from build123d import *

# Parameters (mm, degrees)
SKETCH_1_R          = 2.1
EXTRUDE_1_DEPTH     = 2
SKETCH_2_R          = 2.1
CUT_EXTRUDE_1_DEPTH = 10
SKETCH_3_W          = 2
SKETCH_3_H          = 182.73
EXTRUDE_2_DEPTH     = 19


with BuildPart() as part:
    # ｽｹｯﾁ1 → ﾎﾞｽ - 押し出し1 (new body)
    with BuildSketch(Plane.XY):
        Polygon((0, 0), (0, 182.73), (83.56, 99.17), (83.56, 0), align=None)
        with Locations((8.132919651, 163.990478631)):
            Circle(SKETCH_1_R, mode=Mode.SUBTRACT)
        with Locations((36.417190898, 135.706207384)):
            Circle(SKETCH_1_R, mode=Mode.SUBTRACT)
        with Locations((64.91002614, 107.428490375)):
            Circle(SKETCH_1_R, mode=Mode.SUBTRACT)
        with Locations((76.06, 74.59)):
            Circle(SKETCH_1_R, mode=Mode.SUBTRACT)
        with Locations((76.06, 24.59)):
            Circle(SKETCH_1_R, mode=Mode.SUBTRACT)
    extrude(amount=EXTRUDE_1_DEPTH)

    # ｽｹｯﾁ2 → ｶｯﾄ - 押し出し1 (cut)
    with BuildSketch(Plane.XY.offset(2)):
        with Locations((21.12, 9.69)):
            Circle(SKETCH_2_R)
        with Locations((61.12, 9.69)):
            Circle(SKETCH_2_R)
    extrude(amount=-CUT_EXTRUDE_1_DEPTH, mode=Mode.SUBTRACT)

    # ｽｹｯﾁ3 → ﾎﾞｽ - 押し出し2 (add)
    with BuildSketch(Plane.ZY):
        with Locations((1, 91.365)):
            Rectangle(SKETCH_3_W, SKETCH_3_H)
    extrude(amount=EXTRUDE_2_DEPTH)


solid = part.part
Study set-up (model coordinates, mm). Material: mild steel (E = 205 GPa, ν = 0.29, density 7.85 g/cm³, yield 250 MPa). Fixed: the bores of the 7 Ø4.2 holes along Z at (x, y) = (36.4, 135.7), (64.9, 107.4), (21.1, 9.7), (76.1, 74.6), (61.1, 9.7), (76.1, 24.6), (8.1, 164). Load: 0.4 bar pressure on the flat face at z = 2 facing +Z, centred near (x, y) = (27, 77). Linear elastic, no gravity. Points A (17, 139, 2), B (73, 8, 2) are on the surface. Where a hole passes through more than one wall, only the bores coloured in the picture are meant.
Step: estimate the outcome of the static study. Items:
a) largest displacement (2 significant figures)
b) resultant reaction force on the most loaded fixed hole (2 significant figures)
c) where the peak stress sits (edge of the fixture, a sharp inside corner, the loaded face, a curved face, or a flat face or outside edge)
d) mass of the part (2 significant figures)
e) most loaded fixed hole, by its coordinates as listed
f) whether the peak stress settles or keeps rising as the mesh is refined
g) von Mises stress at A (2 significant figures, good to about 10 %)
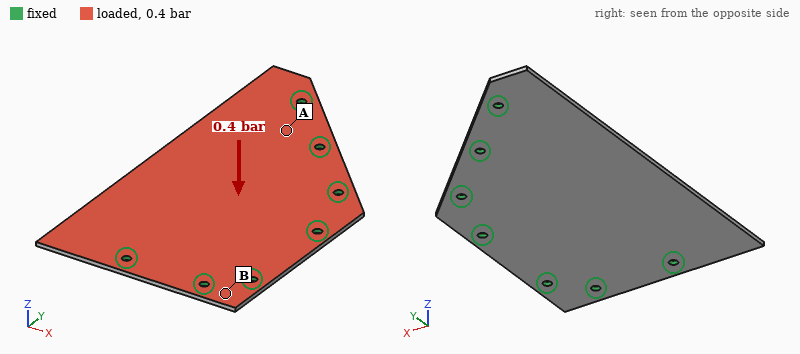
0.48 mm
190 N
edge of the fixture
240 g
(21.1, 9.7)
keeps rising
46 MPa
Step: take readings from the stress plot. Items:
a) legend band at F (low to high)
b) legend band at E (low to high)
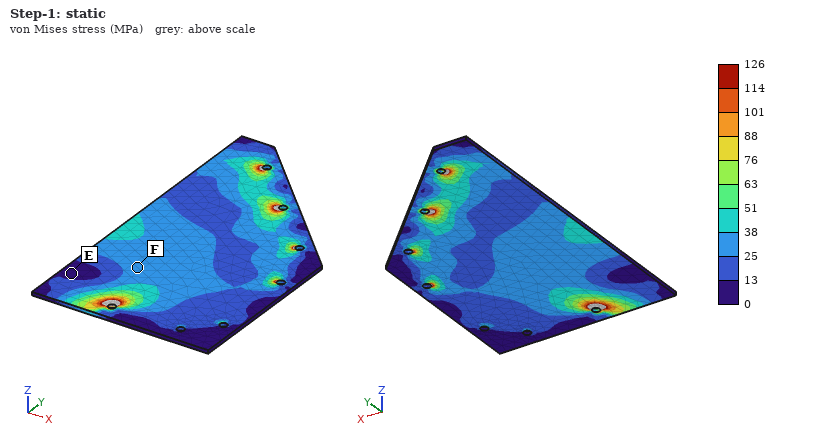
25 to 38 MPa
0 to 13 MPa
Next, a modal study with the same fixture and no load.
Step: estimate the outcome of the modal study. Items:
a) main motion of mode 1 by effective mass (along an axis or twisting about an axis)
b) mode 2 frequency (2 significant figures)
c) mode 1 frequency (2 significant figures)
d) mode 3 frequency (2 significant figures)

along Z
1100 Hz
500 Hz
1300 Hz
